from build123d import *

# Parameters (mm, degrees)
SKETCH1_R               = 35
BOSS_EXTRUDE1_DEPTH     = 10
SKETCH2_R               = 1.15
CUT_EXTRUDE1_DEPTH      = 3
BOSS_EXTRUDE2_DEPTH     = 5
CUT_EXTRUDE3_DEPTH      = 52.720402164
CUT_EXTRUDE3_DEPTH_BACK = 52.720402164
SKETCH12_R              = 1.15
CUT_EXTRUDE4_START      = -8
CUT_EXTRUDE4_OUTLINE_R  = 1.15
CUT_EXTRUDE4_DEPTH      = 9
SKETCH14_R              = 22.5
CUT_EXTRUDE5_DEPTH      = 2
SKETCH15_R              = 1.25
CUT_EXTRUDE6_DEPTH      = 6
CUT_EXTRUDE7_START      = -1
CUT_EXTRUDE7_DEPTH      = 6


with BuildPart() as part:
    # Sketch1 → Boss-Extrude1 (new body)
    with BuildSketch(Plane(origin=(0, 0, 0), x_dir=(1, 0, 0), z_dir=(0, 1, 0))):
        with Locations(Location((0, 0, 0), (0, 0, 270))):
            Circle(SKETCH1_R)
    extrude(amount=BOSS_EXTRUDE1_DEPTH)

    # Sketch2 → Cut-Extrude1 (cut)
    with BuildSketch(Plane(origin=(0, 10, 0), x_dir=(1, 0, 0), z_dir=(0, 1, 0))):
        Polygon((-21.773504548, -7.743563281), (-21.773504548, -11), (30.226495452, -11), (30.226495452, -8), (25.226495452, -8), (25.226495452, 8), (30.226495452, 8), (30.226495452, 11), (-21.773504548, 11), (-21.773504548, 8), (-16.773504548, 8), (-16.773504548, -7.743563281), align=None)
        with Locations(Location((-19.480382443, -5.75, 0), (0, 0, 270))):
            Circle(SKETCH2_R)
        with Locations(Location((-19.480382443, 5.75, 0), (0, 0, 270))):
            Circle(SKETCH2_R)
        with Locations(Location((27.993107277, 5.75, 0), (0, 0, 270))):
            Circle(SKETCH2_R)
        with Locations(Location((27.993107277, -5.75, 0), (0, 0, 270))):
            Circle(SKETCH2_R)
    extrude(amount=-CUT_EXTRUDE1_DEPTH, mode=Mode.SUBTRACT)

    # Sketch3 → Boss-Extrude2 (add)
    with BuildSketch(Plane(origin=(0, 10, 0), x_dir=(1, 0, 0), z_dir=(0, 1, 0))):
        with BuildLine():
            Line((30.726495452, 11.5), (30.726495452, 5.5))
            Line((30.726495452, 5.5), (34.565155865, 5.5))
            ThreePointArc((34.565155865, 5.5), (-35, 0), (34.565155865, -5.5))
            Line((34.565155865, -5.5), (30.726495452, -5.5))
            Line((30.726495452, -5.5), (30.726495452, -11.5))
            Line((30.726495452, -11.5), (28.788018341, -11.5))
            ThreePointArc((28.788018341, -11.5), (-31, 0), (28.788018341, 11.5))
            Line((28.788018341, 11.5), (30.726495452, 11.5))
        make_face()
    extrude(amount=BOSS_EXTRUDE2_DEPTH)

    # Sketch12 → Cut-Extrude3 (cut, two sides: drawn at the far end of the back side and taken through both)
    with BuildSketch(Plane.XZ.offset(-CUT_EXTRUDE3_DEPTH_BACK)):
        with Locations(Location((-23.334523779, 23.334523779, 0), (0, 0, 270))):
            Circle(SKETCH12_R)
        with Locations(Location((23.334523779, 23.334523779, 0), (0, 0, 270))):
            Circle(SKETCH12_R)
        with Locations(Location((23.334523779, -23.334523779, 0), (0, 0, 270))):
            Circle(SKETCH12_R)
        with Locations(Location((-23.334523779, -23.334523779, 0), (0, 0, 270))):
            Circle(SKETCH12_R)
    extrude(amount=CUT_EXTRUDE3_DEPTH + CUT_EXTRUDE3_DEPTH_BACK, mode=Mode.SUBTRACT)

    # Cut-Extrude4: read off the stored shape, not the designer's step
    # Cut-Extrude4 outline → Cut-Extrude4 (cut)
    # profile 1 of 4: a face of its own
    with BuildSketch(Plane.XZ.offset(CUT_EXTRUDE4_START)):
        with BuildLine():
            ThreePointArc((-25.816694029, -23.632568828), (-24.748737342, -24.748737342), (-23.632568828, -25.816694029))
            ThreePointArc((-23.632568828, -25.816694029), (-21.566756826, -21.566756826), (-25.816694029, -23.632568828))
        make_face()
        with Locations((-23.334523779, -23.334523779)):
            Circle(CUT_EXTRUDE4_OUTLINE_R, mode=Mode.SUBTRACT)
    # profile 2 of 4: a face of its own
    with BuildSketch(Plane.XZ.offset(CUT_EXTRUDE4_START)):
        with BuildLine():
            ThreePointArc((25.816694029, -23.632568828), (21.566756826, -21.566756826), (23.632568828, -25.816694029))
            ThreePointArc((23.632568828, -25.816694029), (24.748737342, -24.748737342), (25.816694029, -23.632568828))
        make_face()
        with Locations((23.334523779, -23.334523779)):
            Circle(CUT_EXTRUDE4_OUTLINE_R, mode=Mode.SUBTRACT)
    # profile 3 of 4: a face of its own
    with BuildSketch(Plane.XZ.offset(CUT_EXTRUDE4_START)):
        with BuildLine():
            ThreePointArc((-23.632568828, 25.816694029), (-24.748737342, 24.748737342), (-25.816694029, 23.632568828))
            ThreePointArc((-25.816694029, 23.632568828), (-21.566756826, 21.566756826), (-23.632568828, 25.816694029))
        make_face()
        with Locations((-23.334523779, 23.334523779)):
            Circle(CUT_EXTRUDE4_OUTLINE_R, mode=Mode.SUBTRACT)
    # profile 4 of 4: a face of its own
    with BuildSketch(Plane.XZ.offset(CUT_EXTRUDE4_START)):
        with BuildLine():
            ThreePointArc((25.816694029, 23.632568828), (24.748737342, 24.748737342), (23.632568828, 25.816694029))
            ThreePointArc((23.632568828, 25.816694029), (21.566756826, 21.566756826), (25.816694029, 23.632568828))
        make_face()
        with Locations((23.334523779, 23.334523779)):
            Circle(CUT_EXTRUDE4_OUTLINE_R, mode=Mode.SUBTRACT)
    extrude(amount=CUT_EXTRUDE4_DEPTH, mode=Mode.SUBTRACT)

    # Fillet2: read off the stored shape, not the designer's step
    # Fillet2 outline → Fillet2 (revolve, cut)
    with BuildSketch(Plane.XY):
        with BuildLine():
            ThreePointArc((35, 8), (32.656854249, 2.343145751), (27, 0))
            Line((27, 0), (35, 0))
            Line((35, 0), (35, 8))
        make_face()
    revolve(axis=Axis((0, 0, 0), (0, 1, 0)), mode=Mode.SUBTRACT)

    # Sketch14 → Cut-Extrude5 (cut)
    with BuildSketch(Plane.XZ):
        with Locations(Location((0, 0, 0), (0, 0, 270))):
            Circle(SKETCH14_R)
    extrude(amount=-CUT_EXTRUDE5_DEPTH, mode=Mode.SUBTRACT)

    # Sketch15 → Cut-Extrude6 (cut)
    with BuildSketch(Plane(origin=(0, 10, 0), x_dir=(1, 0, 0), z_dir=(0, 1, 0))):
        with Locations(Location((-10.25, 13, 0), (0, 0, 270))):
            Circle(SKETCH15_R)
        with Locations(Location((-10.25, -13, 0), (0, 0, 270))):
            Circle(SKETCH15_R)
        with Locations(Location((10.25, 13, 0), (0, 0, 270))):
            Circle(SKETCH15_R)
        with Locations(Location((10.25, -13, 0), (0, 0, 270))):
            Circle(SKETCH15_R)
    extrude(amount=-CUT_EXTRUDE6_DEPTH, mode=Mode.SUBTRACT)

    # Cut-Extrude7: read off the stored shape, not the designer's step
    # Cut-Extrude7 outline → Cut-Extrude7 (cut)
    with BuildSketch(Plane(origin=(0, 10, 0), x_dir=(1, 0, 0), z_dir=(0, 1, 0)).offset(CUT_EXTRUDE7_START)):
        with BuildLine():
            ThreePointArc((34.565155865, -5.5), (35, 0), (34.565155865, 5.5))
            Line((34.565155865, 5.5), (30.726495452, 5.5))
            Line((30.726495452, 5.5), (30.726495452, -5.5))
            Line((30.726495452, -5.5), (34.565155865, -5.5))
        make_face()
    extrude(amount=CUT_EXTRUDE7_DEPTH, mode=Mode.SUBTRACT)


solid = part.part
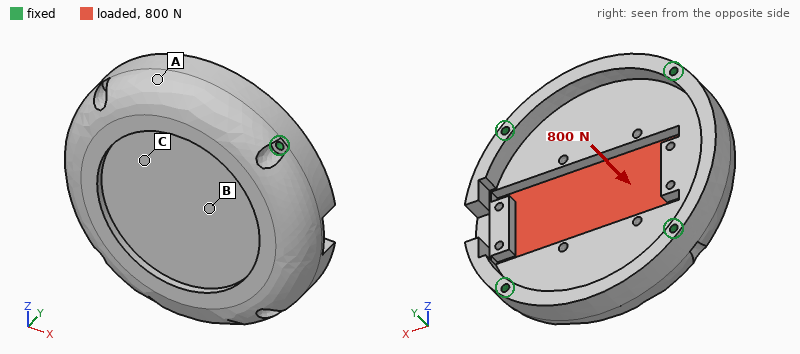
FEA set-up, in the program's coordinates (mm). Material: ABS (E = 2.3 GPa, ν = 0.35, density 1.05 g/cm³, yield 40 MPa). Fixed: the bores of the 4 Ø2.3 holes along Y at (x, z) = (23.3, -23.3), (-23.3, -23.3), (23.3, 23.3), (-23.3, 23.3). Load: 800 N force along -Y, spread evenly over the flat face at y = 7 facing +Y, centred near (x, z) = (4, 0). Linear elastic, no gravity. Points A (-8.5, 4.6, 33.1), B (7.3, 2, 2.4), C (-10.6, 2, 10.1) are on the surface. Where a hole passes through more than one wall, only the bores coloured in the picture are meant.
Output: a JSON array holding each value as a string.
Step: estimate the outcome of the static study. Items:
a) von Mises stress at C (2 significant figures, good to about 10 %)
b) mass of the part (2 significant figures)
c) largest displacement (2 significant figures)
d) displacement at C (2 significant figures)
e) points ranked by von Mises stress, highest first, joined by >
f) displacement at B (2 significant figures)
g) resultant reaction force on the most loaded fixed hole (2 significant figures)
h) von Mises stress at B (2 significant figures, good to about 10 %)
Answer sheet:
["5.1 MPa", "34 g", "0.30 mm", "0.18 mm", "B > C > A", "0.28 mm", "400 N", "11 MPa"]
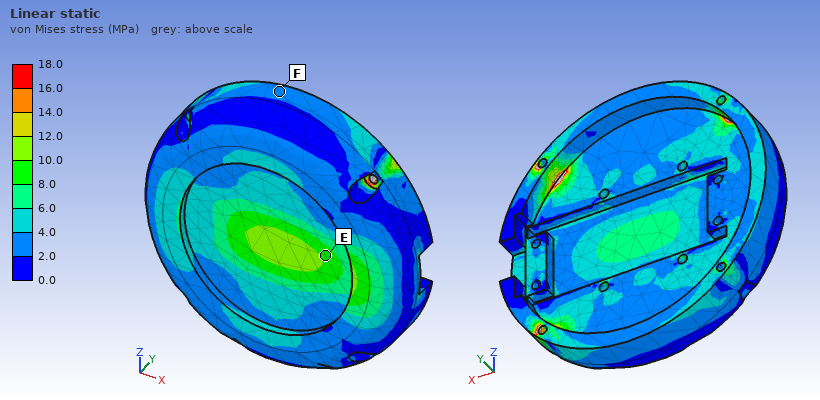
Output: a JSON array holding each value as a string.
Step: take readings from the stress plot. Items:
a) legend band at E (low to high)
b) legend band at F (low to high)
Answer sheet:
["8.0 to 10.0 MPa", "2.0 to 4.0 MPa"]
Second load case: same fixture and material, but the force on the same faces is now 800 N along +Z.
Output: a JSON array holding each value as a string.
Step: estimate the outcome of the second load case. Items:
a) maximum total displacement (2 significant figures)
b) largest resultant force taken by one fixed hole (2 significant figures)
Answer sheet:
["52 µm", "220 N"]
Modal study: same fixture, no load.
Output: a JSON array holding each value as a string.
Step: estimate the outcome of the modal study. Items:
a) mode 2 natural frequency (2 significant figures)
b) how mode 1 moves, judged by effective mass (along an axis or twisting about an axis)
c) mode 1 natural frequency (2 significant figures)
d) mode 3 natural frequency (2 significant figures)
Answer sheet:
["4100 Hz", "along Y", "2900 Hz", "4100 Hz"]
